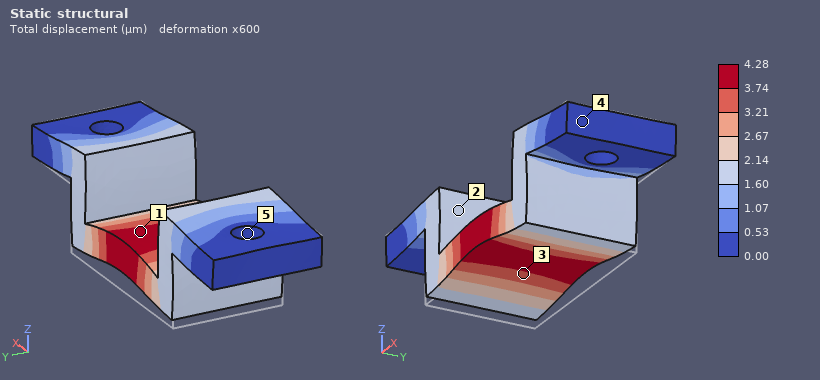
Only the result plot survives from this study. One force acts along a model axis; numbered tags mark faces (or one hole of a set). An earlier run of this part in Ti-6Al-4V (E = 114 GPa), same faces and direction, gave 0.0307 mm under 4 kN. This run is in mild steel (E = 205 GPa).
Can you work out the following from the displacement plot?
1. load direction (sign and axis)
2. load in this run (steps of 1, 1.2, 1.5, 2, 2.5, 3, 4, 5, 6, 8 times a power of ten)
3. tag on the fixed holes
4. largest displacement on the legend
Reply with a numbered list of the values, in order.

1. +Z
2. 1 kN
3. 5
4. 4.28 µm
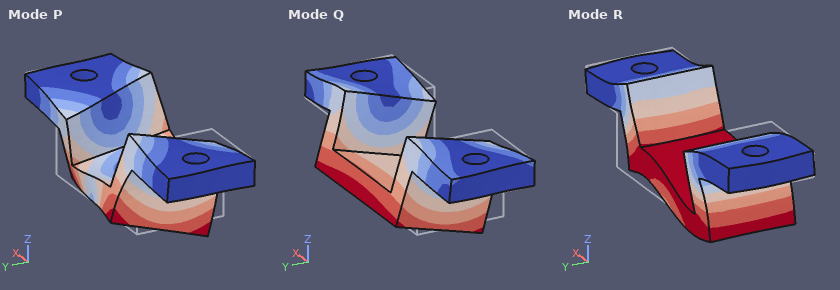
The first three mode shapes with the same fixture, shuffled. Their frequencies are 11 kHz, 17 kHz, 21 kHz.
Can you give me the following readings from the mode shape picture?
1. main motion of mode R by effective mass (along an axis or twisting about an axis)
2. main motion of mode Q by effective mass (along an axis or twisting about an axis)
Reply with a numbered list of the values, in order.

1. along X
2. along Y
